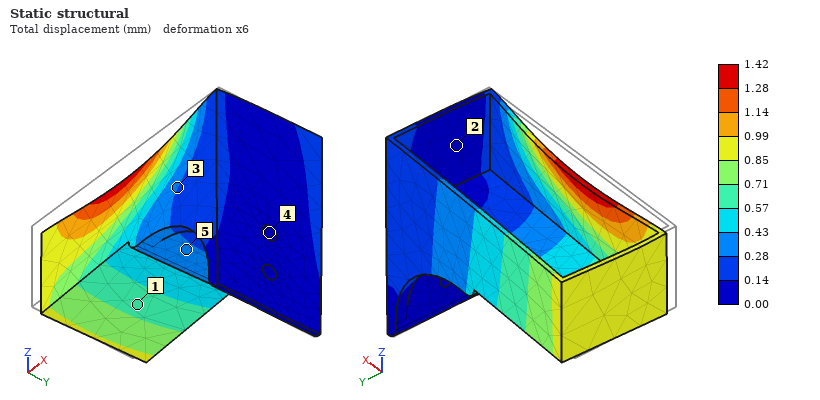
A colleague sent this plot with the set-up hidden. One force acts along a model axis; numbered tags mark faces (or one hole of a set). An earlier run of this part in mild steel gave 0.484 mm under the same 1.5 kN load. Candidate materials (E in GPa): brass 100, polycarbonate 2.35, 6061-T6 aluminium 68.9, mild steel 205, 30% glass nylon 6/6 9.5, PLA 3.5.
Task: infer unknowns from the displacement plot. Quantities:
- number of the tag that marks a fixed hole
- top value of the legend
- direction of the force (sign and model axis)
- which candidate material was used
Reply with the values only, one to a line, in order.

4
1.42 mm
+Y
6061-T6 aluminium
